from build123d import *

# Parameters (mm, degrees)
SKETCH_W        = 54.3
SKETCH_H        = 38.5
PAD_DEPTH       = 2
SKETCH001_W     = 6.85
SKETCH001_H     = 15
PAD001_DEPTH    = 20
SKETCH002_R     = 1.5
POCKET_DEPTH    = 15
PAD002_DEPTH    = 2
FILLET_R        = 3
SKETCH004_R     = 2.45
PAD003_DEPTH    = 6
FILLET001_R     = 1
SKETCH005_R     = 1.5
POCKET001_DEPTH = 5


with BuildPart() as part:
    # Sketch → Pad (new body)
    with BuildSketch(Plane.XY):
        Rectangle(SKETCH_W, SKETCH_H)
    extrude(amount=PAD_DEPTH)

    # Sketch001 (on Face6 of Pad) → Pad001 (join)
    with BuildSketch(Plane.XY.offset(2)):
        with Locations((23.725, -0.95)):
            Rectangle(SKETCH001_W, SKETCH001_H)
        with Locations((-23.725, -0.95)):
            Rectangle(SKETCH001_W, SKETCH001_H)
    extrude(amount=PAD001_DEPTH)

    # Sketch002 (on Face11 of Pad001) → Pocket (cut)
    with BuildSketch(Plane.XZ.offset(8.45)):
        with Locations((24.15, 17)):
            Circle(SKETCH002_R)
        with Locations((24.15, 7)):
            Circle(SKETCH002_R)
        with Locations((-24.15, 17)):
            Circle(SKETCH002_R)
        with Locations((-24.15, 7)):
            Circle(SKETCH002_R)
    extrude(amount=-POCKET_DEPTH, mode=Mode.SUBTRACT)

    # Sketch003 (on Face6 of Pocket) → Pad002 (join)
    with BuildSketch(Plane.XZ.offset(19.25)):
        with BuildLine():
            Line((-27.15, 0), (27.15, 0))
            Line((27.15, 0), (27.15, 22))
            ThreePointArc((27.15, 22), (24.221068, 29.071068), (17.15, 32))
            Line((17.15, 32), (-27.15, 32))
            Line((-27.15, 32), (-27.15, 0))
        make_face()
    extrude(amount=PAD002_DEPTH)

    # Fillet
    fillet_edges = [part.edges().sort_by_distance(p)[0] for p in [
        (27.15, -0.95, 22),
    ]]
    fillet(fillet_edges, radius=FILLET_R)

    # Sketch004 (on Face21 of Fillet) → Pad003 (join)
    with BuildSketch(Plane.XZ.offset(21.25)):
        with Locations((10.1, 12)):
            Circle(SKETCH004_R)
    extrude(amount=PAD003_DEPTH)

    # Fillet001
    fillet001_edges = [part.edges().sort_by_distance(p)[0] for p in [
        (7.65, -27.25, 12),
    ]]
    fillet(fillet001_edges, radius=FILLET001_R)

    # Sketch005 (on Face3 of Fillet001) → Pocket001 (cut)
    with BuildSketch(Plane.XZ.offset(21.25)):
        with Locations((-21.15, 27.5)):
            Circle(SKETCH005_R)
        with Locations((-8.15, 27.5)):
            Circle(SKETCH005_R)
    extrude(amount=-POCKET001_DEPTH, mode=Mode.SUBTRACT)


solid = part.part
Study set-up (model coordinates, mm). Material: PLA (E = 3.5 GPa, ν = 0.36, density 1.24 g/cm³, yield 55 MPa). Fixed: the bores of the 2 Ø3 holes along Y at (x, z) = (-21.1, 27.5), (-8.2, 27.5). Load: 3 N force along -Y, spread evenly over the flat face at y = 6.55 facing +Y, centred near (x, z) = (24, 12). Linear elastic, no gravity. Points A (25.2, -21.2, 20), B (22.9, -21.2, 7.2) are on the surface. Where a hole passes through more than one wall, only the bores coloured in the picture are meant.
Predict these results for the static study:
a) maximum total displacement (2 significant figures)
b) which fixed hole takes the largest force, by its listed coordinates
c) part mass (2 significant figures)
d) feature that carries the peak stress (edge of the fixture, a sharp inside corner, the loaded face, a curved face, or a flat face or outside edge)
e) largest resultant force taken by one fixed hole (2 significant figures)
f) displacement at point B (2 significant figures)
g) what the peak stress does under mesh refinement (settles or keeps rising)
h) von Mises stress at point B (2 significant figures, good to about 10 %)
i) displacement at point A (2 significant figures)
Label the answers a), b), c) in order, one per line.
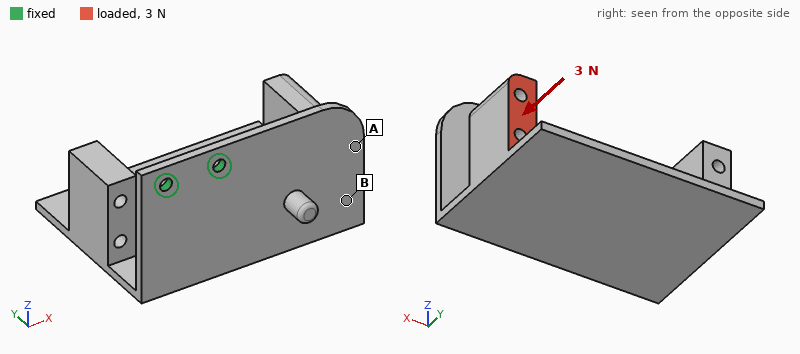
a) 0.78 mm
b) (-8.2, 27.5)
c) 14 g
d) edge of the fixture
e) 7.2 N
f) 0.49 mm
g) keeps rising
h) 0.89 MPa
i) 0.38 mm
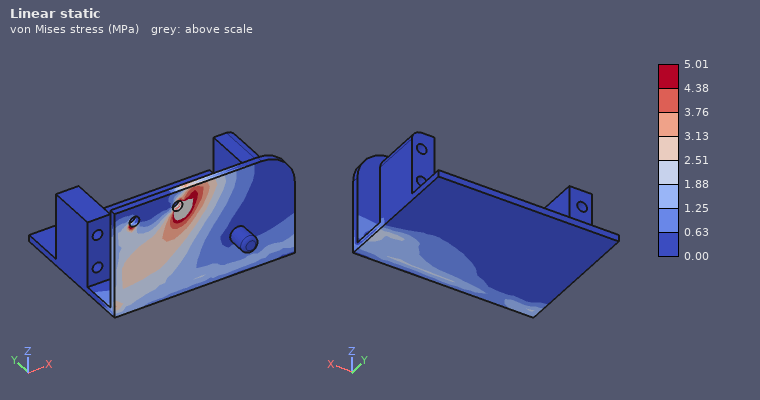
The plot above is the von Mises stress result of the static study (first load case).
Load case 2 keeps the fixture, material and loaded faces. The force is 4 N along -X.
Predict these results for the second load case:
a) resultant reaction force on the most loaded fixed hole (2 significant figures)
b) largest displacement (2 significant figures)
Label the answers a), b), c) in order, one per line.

a) 7.2 N
b) 0.86 mm
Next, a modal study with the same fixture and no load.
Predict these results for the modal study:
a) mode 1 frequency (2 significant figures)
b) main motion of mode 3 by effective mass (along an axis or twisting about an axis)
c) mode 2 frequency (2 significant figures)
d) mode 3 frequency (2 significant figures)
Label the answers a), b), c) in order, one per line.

a) 110 Hz
b) along Y
c) 150 Hz
d) 300 Hz
